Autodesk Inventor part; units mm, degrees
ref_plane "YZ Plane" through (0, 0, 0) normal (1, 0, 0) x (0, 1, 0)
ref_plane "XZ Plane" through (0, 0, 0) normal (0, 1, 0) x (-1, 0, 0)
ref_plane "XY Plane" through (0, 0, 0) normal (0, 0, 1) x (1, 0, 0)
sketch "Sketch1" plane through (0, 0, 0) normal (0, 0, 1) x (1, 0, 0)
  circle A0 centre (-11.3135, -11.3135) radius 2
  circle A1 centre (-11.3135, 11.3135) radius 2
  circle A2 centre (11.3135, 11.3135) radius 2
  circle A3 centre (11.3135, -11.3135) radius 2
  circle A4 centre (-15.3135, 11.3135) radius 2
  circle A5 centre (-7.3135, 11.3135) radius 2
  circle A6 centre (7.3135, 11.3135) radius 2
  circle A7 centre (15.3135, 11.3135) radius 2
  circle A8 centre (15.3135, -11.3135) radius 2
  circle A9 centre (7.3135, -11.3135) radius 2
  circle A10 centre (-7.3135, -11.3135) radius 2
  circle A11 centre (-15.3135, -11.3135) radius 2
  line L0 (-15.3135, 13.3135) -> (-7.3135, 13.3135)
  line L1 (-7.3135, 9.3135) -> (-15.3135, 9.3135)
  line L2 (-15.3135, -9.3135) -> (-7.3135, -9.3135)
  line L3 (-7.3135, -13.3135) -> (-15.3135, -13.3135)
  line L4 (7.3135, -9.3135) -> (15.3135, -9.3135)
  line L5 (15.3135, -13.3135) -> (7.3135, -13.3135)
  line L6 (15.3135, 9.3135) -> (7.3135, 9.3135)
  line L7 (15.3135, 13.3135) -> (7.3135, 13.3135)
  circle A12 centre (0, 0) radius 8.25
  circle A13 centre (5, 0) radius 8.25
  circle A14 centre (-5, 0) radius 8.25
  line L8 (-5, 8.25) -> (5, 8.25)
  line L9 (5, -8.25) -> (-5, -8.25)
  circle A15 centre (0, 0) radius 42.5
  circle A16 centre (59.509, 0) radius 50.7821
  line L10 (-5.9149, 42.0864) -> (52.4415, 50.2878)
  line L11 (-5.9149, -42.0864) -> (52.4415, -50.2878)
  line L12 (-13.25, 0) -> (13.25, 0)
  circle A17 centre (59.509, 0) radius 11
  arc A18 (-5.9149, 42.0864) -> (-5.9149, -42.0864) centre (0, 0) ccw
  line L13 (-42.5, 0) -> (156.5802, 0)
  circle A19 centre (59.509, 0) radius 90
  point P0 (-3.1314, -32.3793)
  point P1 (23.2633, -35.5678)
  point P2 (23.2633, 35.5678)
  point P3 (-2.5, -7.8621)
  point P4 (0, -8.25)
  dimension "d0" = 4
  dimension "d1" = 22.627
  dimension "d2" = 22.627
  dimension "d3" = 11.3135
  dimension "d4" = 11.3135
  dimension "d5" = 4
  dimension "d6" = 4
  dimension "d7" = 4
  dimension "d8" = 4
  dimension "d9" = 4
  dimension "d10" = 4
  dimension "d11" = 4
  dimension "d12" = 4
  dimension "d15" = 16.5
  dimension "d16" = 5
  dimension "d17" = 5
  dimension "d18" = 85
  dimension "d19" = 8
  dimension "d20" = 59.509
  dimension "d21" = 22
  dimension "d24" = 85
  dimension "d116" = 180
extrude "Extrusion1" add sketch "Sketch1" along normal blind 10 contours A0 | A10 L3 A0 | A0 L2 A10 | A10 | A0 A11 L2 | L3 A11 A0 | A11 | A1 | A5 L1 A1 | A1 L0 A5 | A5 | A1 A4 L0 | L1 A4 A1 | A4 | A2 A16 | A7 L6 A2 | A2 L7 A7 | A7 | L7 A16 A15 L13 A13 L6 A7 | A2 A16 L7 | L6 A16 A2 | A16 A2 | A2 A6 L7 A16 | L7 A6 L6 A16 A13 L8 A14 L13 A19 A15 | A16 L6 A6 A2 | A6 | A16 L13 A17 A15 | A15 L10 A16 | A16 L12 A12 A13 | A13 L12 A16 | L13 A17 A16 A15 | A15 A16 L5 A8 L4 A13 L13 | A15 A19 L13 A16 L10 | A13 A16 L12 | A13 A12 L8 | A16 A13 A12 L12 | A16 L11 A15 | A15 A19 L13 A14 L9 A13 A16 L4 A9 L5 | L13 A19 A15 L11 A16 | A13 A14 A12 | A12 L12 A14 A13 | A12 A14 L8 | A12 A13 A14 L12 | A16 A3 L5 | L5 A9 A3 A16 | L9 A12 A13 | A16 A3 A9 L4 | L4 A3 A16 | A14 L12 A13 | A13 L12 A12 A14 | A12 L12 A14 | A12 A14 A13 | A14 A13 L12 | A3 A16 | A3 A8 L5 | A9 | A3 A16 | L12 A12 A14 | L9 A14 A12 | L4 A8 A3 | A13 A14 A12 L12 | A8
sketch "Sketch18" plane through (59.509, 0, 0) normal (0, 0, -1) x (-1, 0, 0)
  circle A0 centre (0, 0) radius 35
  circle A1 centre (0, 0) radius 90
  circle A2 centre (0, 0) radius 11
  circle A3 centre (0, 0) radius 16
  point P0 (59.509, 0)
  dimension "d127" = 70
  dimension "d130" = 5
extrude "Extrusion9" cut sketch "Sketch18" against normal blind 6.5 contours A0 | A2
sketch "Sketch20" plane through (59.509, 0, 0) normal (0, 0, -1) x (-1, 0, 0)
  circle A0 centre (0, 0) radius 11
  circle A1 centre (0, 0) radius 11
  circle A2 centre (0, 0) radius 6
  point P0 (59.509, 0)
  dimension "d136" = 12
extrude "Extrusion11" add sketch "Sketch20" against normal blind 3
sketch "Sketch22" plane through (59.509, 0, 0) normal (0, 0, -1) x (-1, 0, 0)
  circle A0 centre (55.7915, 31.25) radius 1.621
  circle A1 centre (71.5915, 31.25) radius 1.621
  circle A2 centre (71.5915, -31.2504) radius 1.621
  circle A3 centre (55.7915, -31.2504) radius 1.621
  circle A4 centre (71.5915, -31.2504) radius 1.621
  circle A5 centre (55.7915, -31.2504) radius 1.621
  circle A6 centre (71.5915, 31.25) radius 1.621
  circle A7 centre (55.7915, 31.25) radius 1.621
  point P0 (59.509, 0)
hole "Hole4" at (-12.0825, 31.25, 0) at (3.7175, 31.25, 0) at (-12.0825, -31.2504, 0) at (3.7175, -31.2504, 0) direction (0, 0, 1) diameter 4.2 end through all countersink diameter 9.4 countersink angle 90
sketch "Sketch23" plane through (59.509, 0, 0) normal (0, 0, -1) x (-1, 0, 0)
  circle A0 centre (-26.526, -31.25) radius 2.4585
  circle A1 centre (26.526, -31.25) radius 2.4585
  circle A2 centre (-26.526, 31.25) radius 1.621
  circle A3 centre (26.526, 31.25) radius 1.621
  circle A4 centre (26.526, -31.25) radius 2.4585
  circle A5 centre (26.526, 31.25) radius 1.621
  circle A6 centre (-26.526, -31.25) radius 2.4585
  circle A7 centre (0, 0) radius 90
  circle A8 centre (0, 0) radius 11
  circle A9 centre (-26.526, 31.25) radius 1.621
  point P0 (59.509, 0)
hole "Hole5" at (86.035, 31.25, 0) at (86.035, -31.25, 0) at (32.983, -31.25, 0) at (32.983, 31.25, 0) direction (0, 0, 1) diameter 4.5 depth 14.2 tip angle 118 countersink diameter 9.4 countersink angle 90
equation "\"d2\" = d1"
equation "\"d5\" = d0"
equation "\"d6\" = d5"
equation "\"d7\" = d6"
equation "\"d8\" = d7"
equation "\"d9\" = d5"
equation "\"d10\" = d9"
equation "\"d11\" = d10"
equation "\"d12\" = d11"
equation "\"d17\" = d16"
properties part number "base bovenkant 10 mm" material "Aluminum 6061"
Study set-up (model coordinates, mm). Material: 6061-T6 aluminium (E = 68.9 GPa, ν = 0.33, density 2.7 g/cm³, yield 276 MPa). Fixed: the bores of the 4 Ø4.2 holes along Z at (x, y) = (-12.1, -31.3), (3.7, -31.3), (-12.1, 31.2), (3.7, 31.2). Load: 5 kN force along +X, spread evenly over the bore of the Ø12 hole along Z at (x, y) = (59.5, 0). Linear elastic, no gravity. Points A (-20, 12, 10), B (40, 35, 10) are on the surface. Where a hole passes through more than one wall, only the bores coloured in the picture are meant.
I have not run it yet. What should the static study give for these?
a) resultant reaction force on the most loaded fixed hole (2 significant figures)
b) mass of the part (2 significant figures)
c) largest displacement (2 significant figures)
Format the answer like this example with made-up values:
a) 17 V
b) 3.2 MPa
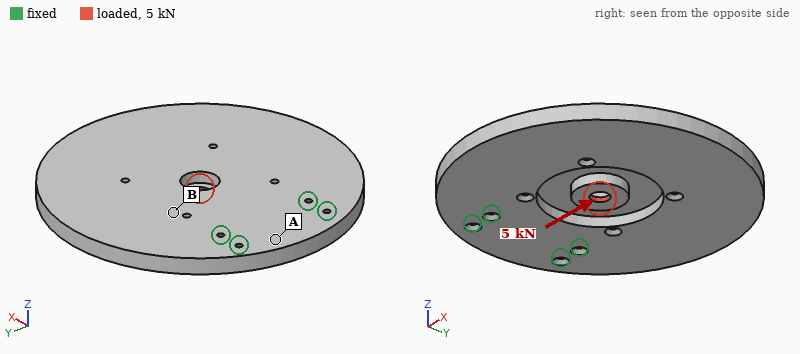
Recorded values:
a) 1.6 kN
b) 620 g
c) 0.29 mm
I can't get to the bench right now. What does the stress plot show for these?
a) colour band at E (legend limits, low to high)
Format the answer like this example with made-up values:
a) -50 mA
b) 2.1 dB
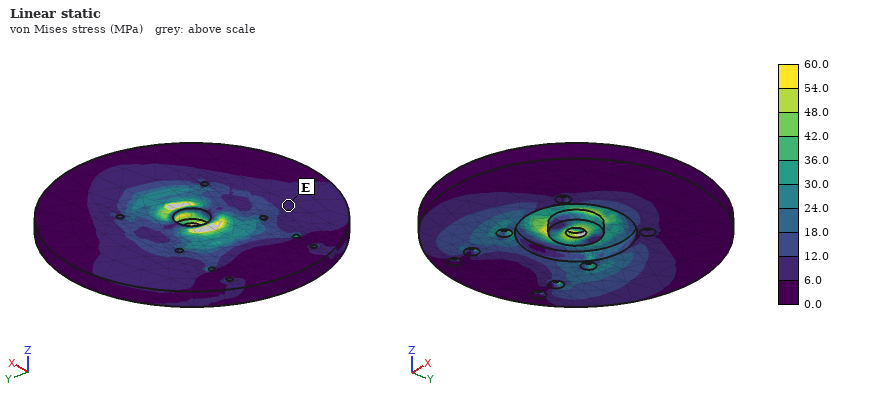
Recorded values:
a) 6.0 to 12.0 MPa
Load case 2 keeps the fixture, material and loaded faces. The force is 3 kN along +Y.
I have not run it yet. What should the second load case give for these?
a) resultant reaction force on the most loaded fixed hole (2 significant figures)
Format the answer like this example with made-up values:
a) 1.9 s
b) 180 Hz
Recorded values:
a) 2.4 kN
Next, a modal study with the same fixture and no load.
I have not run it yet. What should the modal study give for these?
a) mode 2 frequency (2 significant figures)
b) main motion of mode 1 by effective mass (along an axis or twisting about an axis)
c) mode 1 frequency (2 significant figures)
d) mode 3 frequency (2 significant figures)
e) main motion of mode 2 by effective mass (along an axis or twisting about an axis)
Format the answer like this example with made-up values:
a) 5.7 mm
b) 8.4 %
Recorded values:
a) 750 Hz
b) along Z
c) 360 Hz
d) 1600 Hz
e) twisting about X
